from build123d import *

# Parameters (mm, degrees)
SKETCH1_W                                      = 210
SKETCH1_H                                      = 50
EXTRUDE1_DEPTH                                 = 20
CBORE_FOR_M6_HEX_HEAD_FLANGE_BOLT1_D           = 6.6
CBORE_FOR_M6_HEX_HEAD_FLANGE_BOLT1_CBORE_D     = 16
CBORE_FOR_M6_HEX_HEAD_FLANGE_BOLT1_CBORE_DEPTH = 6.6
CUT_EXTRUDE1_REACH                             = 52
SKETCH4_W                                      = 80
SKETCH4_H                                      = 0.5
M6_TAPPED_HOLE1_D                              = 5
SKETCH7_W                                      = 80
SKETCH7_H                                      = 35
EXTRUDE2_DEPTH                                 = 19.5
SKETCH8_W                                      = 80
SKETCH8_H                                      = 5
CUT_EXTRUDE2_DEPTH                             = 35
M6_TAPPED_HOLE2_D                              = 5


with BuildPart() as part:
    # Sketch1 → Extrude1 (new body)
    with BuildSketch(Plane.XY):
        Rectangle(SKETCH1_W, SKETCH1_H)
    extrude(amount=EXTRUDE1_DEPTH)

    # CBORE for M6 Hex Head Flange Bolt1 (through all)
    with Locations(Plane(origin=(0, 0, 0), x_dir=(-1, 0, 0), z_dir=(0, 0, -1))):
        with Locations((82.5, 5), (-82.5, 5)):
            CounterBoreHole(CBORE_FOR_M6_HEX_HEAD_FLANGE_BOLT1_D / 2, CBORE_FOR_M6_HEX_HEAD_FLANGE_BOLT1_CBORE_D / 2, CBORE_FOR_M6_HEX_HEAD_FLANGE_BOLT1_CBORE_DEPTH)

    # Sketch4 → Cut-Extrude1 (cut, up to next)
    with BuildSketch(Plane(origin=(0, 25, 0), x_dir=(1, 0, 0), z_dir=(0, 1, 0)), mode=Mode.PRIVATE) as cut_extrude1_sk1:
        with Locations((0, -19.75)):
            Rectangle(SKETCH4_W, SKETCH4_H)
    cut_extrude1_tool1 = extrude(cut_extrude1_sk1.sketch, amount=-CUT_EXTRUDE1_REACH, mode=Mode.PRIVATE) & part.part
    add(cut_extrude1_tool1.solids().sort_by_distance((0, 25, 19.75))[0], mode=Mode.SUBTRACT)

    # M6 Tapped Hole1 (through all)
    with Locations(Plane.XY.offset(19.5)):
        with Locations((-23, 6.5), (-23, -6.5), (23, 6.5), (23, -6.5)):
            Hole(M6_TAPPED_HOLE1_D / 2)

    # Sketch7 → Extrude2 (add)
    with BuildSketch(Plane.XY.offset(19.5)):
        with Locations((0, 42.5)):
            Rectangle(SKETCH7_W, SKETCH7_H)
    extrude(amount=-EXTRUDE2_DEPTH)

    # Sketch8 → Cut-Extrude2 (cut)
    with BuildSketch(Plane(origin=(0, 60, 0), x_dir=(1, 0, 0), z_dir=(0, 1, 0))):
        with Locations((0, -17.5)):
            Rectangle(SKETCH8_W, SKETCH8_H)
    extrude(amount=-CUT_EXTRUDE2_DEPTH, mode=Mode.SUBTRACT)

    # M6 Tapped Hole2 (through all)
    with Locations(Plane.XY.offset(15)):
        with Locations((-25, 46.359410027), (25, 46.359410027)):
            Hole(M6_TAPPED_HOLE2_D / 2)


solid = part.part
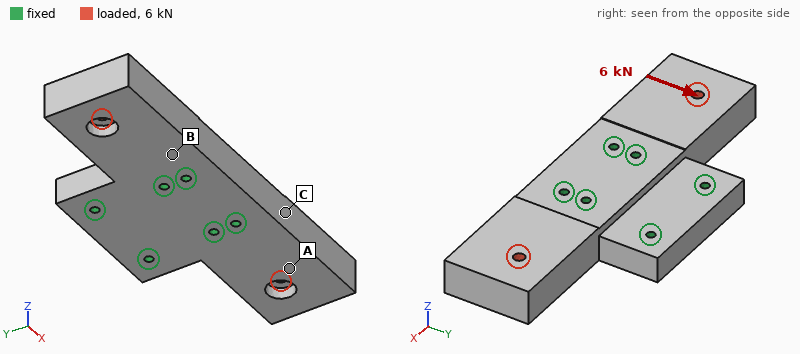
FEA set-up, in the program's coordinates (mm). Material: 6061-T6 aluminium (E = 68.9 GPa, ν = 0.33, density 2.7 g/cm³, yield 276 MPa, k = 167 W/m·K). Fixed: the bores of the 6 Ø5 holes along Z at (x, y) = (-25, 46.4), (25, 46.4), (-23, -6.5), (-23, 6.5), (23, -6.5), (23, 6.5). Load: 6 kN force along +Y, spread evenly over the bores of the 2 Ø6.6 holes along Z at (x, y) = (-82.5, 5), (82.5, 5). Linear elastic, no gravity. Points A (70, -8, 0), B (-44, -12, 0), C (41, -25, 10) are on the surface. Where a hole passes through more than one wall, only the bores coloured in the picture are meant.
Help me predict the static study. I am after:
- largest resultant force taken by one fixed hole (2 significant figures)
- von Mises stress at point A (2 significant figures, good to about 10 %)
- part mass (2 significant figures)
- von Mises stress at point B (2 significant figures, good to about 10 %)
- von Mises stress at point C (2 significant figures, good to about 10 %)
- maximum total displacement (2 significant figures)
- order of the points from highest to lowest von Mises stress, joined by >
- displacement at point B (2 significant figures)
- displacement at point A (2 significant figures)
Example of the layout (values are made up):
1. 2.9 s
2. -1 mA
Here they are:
1. 3.0 kN
2. 3.6 MPa
3. 660 g
4. 7.9 MPa
5. 13 MPa
6. 39 µm
7. C > B > A
8. 6.7 µm
9. 17 µm
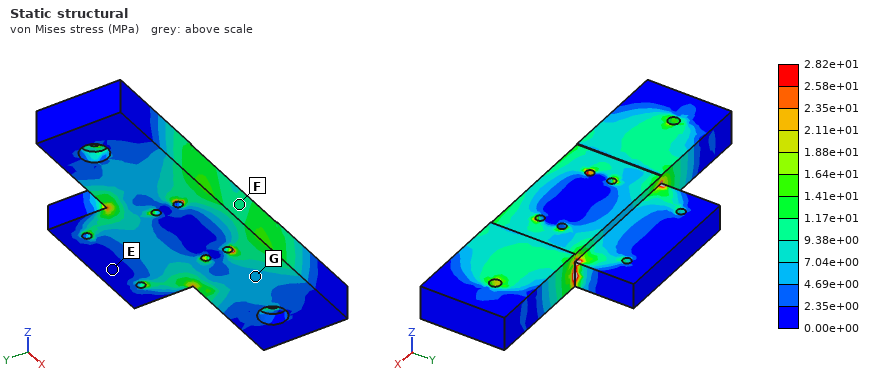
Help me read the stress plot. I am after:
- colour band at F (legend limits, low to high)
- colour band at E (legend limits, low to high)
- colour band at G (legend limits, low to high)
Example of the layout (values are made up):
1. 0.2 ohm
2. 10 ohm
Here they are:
1. 9.38e+00 to 1.17e+01 MPa
2. 0.00e+00 to 2.35e+00 MPa
3. 4.69e+00 to 7.04e+00 MPa
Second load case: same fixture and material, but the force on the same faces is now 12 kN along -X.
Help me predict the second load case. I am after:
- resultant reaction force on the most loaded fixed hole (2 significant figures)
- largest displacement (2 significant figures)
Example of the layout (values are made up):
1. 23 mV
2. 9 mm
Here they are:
1. 2.9 kN
2. 33 µm
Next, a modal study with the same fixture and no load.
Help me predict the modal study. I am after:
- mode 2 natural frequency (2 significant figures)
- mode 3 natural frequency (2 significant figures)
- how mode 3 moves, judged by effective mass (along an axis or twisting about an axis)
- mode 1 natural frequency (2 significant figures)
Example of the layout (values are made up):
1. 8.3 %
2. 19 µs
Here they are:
1. 2300 Hz
2. 4500 Hz
3. twisting about Z
4. 2300 Hz
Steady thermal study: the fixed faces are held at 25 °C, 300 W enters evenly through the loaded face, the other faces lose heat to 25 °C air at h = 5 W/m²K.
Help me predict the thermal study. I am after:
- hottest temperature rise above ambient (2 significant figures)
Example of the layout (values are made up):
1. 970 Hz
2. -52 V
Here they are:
1. 70 K
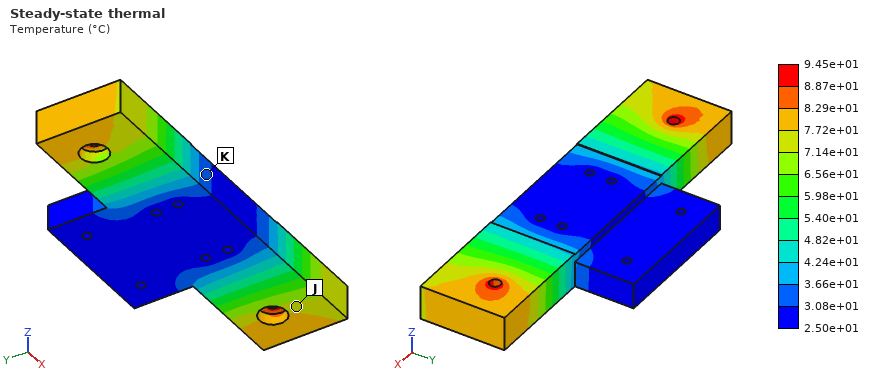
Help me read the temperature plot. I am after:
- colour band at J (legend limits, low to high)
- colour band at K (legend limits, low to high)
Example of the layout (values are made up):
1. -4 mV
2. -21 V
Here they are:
1. 7.14e+01 to 7.72e+01 °C
2. 3.08e+01 to 3.66e+01 °C
